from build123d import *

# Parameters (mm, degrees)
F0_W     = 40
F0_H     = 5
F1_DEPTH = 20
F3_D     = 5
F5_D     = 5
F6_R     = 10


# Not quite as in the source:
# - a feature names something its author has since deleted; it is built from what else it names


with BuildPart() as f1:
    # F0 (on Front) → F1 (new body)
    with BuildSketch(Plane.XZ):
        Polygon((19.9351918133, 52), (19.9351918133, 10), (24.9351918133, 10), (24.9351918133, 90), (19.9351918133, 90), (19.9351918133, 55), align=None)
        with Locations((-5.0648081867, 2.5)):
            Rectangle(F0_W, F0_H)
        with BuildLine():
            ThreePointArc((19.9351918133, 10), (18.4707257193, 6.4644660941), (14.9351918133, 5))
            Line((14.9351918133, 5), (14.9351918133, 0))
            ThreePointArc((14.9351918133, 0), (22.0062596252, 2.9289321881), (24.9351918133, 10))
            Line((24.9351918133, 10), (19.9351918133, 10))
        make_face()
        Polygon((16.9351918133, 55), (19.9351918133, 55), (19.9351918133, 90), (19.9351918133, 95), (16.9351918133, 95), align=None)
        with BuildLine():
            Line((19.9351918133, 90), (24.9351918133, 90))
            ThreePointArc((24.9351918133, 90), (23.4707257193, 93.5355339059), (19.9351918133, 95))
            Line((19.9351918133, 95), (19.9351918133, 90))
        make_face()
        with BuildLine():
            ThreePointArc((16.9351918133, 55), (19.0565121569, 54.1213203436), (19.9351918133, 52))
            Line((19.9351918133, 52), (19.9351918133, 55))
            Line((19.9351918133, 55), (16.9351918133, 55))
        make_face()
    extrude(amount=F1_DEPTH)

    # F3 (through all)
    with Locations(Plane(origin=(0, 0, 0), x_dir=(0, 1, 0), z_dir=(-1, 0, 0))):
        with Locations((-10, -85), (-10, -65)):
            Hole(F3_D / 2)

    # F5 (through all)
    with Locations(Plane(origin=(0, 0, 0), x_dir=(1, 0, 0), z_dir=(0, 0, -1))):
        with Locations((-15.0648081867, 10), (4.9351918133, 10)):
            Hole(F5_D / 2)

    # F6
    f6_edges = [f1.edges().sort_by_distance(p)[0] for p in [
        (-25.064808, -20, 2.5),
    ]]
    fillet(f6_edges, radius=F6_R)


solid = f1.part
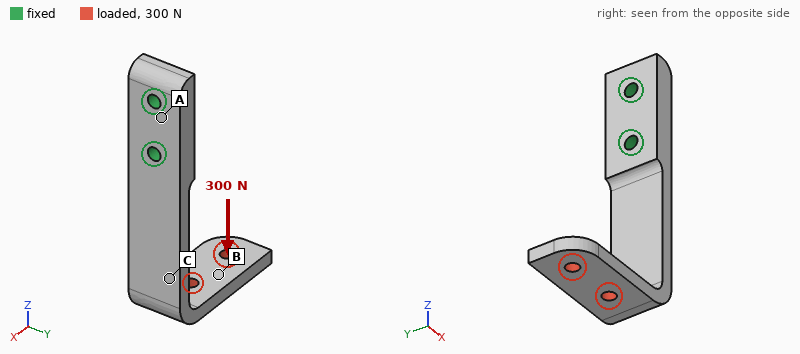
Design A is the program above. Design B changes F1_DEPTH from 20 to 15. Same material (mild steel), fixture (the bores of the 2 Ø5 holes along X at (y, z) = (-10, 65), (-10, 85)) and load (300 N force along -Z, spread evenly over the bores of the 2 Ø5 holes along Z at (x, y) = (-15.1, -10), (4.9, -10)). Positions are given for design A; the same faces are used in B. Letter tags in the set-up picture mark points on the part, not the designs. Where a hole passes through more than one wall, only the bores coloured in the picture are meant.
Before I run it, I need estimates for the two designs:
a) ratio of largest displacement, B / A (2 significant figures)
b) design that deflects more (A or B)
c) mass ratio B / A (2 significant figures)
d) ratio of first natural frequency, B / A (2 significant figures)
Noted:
1.3
B
0.74
1.0
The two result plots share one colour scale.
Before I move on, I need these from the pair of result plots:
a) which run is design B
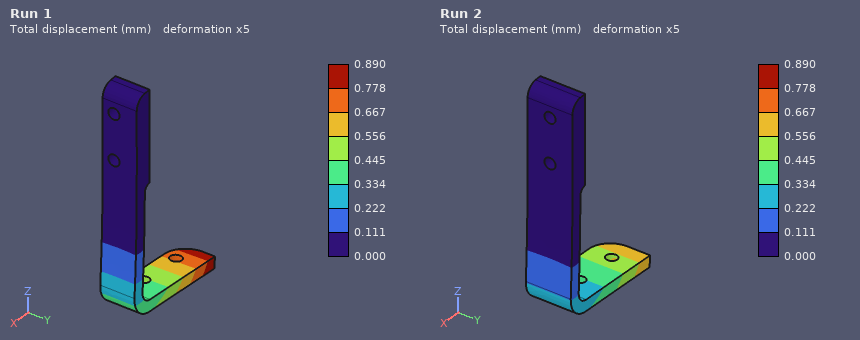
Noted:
Run 1
